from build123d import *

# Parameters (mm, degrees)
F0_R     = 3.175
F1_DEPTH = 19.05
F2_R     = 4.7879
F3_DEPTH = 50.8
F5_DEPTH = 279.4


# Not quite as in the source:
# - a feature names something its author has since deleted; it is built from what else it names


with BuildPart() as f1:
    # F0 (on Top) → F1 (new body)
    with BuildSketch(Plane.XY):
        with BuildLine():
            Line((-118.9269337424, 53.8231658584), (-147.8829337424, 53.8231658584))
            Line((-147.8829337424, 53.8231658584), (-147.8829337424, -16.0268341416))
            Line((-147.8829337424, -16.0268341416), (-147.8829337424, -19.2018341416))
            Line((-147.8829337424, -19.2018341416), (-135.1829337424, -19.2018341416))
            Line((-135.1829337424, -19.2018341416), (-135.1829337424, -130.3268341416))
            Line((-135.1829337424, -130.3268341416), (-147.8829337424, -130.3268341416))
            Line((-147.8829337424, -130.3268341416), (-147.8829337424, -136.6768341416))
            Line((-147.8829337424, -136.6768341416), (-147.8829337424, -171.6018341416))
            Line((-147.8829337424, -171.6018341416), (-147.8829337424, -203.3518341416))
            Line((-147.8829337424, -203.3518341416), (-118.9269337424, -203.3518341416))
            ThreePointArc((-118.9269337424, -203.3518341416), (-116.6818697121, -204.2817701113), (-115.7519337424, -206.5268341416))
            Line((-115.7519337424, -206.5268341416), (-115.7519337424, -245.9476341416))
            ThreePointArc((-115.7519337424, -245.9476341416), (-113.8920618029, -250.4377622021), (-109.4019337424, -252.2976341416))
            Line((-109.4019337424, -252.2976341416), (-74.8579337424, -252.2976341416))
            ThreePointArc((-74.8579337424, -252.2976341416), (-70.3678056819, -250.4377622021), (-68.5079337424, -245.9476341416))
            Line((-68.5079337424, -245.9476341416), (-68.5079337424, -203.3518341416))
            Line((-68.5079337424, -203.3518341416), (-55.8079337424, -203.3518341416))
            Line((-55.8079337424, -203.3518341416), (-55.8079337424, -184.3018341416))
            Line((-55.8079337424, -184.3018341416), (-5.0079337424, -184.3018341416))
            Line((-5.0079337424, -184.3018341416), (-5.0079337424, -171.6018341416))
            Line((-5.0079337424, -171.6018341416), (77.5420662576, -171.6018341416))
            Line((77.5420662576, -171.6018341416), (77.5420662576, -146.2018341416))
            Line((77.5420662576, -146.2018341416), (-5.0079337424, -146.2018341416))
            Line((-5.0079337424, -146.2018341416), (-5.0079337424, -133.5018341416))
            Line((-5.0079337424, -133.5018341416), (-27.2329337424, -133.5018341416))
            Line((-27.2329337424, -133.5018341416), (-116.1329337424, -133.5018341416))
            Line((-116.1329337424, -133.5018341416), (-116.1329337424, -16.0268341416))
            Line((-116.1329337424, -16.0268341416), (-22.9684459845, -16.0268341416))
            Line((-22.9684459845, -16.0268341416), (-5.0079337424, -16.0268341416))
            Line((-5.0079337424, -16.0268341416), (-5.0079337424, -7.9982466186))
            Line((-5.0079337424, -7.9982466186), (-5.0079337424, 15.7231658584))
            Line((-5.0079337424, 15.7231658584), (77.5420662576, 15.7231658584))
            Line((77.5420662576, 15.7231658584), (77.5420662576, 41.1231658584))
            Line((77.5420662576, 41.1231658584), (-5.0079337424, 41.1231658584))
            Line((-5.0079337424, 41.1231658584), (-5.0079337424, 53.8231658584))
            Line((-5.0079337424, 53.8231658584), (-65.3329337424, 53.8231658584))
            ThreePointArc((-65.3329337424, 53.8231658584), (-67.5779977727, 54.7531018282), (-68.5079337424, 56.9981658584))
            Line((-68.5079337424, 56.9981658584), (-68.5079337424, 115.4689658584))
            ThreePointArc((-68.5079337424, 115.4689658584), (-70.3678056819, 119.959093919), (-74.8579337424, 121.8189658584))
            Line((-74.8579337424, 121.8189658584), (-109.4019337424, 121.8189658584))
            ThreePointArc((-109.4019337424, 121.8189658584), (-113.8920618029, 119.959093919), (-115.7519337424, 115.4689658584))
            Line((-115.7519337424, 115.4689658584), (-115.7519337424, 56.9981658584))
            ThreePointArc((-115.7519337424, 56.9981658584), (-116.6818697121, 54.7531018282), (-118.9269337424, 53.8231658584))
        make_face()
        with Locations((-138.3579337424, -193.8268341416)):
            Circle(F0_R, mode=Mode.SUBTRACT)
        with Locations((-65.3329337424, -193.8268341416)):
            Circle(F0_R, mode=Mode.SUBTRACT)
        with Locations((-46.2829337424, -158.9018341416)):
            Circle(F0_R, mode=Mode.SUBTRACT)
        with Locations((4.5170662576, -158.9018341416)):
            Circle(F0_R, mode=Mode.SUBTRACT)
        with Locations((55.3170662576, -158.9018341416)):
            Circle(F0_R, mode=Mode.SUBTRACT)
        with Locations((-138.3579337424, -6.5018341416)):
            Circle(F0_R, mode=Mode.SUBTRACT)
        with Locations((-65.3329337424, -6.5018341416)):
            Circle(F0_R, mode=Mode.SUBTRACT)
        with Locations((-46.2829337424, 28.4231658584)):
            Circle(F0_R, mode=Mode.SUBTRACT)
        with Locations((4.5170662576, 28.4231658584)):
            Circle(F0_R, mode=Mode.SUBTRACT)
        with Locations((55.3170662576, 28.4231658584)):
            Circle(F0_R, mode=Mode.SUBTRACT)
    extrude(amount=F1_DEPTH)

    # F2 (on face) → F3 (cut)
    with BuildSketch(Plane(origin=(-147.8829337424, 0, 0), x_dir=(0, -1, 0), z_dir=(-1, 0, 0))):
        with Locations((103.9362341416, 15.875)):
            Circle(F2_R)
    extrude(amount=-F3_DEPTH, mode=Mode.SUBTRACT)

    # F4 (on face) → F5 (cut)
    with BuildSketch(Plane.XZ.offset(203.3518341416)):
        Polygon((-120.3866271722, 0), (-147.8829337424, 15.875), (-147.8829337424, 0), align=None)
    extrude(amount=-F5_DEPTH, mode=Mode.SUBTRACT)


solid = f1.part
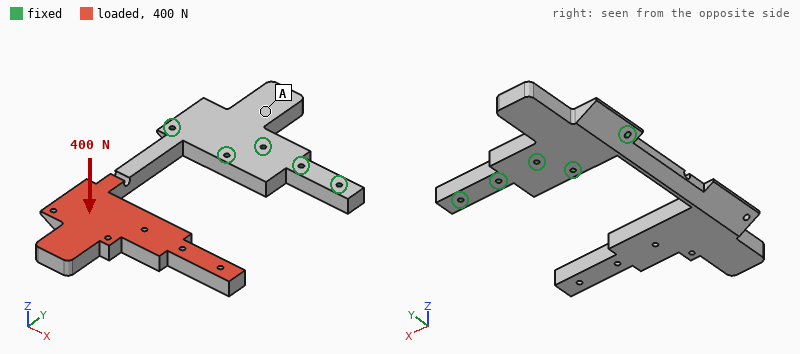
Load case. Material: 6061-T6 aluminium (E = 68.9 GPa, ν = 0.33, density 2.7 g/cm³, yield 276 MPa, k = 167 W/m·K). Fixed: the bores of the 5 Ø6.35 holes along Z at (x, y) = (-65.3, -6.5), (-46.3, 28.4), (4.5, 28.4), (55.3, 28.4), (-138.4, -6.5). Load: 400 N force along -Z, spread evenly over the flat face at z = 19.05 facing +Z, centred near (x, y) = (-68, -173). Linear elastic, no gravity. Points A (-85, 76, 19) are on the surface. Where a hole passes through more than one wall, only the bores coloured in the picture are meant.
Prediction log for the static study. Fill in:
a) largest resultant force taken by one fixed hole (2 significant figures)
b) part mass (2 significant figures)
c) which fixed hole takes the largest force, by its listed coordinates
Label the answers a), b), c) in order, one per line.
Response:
a) 1.3 kN
b) 1.5 kg
c) (-65.3, -6.5)
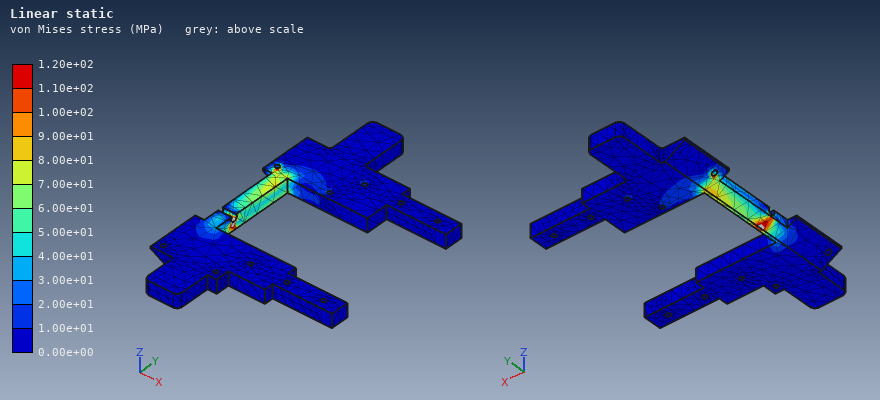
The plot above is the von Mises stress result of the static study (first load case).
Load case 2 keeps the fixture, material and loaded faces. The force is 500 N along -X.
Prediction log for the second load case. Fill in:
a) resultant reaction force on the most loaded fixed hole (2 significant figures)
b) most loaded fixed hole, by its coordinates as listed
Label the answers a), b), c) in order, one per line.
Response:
a) 1.5 kN
b) (-138.4, -6.5)
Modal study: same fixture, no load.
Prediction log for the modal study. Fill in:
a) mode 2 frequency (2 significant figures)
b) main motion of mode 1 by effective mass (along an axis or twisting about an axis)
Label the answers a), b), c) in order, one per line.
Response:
a) 94 Hz
b) along Z
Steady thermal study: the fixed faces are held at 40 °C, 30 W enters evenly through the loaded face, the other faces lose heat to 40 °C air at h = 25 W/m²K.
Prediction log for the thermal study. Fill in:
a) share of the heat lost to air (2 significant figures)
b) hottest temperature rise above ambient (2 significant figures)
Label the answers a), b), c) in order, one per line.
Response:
a) 73 %
b) 30 K
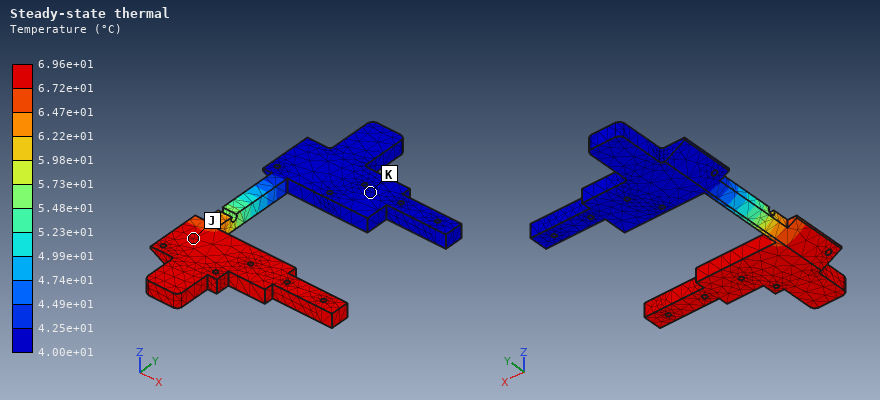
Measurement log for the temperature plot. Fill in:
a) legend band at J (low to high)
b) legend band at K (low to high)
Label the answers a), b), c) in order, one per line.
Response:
a) 6.72e+01 to 6.96e+01 °C
b) 4.00e+01 to 4.25e+01 °C
